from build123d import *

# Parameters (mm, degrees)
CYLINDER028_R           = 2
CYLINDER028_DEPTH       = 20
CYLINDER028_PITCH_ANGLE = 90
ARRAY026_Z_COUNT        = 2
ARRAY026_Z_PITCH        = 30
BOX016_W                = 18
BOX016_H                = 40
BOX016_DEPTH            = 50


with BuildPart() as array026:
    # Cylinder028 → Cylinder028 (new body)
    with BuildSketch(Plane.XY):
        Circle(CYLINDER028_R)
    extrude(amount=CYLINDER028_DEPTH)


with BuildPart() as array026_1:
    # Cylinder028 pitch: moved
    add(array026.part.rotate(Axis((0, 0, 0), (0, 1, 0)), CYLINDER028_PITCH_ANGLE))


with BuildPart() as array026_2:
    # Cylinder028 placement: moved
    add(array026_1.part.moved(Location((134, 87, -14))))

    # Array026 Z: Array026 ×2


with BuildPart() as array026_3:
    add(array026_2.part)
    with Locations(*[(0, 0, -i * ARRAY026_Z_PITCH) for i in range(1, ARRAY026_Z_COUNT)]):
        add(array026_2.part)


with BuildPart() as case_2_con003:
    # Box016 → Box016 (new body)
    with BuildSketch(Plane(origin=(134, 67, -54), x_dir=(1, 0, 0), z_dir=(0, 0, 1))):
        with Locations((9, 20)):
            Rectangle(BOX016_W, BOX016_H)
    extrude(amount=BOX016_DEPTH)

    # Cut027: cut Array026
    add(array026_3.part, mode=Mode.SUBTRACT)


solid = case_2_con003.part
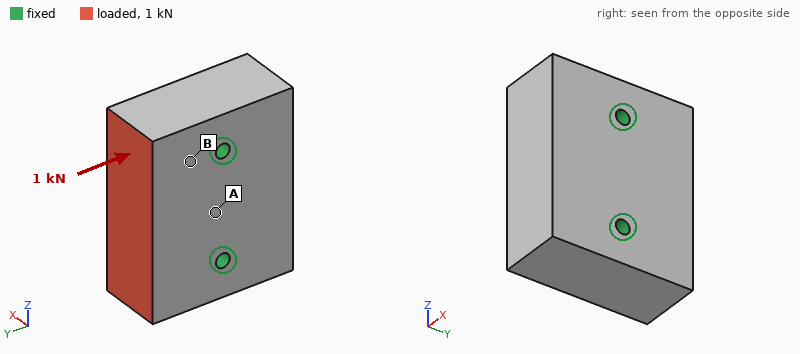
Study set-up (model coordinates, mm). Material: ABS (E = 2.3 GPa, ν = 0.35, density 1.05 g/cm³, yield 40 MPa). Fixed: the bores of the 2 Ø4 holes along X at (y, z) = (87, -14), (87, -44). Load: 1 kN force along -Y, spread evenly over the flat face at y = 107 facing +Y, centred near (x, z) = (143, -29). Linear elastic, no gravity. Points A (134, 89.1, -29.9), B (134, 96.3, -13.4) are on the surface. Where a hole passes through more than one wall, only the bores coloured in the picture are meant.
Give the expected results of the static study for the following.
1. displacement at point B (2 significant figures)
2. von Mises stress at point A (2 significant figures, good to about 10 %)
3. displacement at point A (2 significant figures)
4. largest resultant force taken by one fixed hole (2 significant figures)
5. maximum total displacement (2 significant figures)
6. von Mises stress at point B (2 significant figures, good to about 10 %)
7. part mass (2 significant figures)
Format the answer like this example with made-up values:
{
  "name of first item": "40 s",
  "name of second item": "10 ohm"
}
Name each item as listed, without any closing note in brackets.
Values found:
{
  "displacement at point B": "6.9 µm",
  "von Mises stress at point A": "0.46 MPa",
  "displacement at point A": "7.3 µm",
  "largest resultant force taken by one fixed hole": "500 N",
  "maximum total displacement": "14 µm",
  "von Mises stress at point B": "1.5 MPa",
  "part mass": "37 g"
}
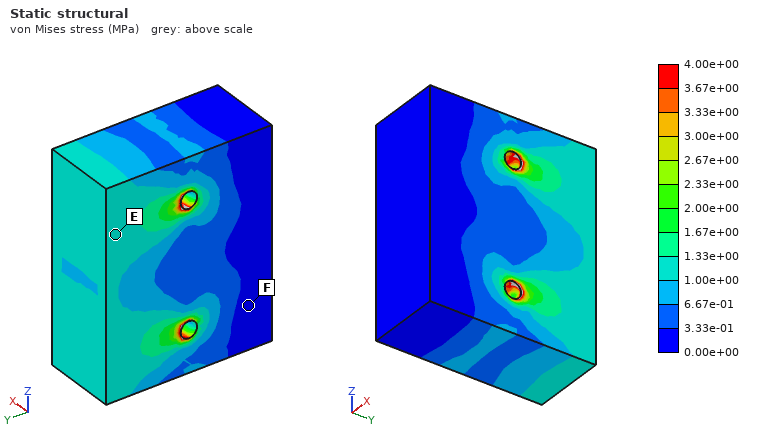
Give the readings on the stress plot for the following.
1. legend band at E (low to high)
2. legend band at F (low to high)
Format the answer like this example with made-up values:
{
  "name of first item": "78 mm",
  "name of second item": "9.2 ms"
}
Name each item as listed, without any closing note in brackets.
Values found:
{
  "legend band at E": "1.00e+00 to 1.33e+00 MPa",
  "legend band at F": "0.00e+00 to 3.33e-01 MPa"
}
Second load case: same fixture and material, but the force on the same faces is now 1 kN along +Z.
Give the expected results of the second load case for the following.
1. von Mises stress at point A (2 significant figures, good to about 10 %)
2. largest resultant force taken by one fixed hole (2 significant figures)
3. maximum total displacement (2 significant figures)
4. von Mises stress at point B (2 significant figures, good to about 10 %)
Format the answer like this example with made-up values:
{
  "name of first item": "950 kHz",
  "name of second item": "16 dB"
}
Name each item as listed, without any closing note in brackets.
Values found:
{
  "von Mises stress at point A": "1.8 MPa",
  "largest resultant force taken by one fixed hole": "790 N",
  "maximum total displacement": "64 µm",
  "von Mises stress at point B": "1.7 MPa"
}
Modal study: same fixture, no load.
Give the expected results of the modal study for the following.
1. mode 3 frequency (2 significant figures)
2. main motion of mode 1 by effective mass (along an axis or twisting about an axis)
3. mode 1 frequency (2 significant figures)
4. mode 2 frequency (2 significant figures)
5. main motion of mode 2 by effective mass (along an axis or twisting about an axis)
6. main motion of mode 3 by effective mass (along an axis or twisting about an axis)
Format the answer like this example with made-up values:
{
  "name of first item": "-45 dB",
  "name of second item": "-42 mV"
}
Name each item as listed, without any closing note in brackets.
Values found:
{
  "mode 3 frequency": "7500 Hz",
  "main motion of mode 1 by effective mass": "twisting about Z",
  "mode 1 frequency": "5100 Hz",
  "mode 2 frequency": "6700 Hz",
  "main motion of mode 2 by effective mass": "along X",
  "main motion of mode 3 by effective mass": "twisting about X"
}
